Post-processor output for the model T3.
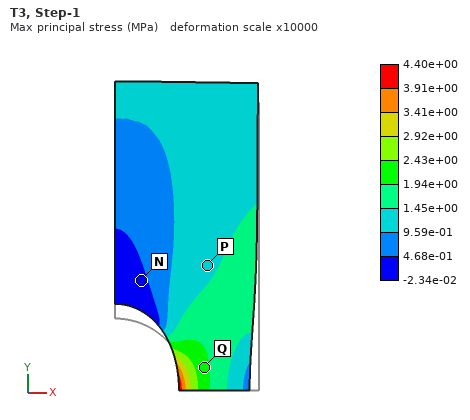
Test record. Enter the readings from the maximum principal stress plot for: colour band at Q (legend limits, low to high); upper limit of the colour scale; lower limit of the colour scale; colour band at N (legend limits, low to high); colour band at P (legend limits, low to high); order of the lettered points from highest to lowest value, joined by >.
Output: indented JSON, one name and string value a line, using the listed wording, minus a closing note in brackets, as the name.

{
  "colour band at Q": "1.94e+00 to 2.43e+00 MPa",
  "upper limit of the colour scale": "4.40e+00 MPa",
  "lower limit of the colour scale": "-2.34e-02 MPa",
  "colour band at N": "-2.34e-02 to 4.68e-01 MPa",
  "colour band at P": "9.59e-01 to 1.45e+00 MPa",
  "order of the lettered points from highest to lowest value, joined by >": "Q > P > N"
}
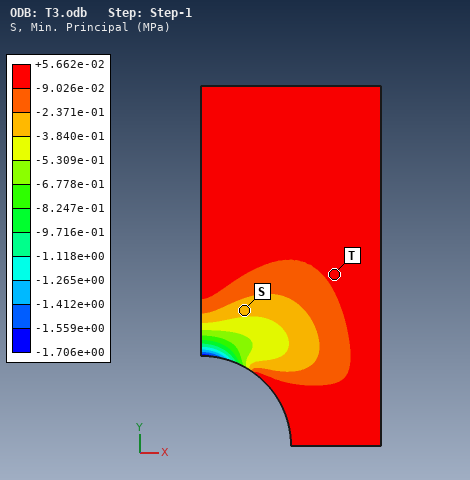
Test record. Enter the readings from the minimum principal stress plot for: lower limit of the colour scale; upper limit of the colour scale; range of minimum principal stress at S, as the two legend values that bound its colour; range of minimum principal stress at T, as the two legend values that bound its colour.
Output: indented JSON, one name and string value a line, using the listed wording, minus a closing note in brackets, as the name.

{
  "lower limit of the colour scale": "-1.706e+00 MPa",
  "upper limit of the colour scale": "+5.662e-02 MPa",
  "range of minimum principal stress at S, as the two legend values that bound its colour": "-3.840e-01 to -2.371e-01 MPa",
  "range of minimum principal stress at T, as the two legend values that bound its colour": "-9.026e-02 to +5.662e-02 MPa"
}
